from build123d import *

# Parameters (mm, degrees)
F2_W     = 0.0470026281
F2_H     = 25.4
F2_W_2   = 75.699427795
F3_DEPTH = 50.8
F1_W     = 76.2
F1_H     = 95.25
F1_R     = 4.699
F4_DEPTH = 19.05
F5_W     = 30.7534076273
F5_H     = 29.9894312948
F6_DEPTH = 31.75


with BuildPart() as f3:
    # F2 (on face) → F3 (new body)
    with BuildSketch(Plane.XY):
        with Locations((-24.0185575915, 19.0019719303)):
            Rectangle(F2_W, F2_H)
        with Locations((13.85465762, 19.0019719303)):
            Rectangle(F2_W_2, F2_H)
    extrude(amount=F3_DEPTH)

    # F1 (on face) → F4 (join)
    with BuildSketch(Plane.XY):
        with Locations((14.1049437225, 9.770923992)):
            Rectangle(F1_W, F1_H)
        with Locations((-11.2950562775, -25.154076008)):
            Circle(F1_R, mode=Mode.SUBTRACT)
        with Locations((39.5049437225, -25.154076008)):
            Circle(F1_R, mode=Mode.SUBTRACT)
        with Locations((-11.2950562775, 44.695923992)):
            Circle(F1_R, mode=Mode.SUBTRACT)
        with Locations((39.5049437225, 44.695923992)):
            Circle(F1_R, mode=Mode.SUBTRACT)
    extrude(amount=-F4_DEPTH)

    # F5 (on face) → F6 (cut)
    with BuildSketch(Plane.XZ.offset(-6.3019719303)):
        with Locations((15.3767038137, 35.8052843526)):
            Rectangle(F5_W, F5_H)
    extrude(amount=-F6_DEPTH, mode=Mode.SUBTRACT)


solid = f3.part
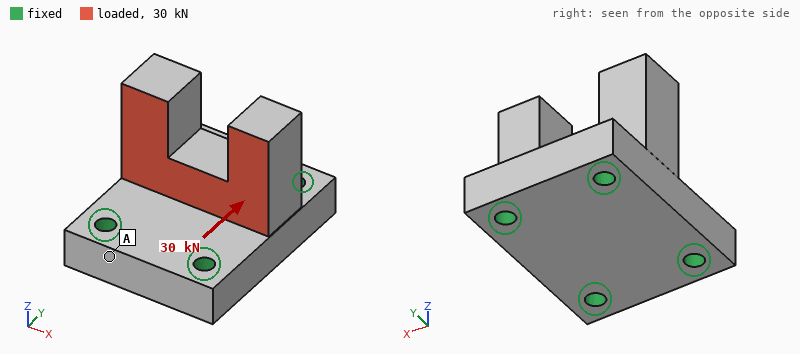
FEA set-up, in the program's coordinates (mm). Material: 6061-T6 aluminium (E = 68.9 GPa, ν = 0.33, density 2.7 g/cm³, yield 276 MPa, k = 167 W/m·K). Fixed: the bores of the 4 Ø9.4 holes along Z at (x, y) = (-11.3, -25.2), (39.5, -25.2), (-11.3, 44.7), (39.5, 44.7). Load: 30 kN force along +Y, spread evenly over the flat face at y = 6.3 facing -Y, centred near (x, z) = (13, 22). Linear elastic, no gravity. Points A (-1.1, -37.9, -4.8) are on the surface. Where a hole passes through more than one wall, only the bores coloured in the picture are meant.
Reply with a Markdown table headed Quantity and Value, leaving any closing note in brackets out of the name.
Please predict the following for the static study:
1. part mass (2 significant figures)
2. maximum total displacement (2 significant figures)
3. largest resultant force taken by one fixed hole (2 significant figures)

| Quantity | Value |
|---|---|
| part mass | 560 g |
| maximum total displacement | 0.19 mm |
| largest resultant force taken by one fixed hole | 12 kN |
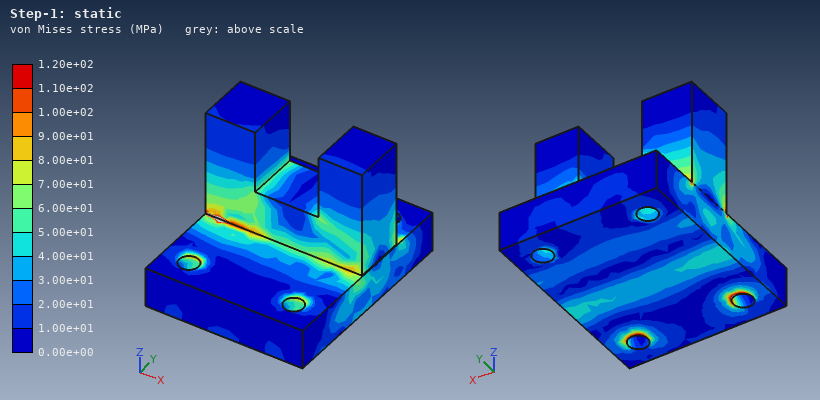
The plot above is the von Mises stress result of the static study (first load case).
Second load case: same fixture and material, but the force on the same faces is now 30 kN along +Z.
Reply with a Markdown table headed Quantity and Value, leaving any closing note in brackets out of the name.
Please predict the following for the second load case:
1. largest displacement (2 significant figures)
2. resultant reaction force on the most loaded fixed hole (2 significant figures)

| Quantity | Value |
|---|---|
| largest displacement | 0.13 mm |
| resultant reaction force on the most loaded fixed hole | 8.8 kN |
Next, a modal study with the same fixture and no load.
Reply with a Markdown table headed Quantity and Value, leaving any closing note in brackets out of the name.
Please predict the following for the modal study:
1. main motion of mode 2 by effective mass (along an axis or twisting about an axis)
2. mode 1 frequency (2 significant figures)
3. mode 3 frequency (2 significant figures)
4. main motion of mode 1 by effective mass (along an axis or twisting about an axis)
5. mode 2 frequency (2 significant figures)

| Quantity | Value |
|---|---|
| main motion of mode 2 by effective mass | along X |
| mode 1 frequency | 5600 Hz |
| mode 3 frequency | 6700 Hz |
| main motion of mode 1 by effective mass | along Y |
| mode 2 frequency | 5900 Hz |
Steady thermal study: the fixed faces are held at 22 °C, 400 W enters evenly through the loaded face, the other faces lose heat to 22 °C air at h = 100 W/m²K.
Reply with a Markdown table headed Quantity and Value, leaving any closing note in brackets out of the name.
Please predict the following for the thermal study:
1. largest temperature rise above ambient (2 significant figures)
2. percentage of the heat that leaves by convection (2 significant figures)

| Quantity | Value |
|---|---|
| largest temperature rise above ambient | 62 K |
| percentage of the heat that leaves by convection | 13 % |
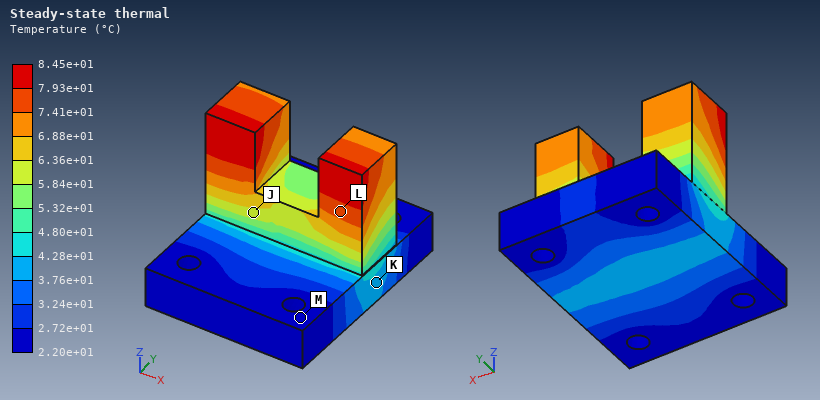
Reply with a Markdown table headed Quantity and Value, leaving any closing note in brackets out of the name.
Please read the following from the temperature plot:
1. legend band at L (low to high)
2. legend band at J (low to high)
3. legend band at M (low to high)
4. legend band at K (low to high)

| Quantity | Value |
|---|---|
| legend band at L | 7.41e+01 to 7.93e+01 °C |
| legend band at J | 5.84e+01 to 6.36e+01 °C |
| legend band at M | 2.20e+01 to 2.72e+01 °C |
| legend band at K | 3.76e+01 to 4.28e+01 °C |
